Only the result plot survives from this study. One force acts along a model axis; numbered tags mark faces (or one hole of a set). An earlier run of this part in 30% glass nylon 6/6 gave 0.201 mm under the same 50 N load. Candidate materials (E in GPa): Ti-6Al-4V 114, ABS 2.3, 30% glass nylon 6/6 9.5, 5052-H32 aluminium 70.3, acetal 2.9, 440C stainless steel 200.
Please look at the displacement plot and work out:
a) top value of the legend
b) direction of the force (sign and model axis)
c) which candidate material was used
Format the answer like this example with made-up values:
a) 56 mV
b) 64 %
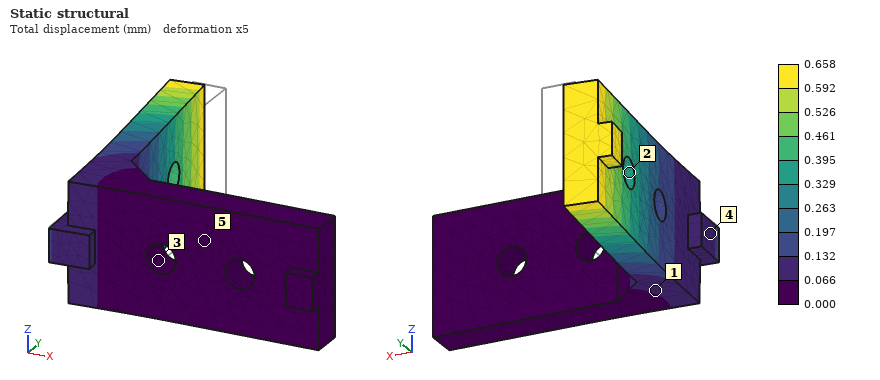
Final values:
a) 0.658 mm
b) -X
c) acetal
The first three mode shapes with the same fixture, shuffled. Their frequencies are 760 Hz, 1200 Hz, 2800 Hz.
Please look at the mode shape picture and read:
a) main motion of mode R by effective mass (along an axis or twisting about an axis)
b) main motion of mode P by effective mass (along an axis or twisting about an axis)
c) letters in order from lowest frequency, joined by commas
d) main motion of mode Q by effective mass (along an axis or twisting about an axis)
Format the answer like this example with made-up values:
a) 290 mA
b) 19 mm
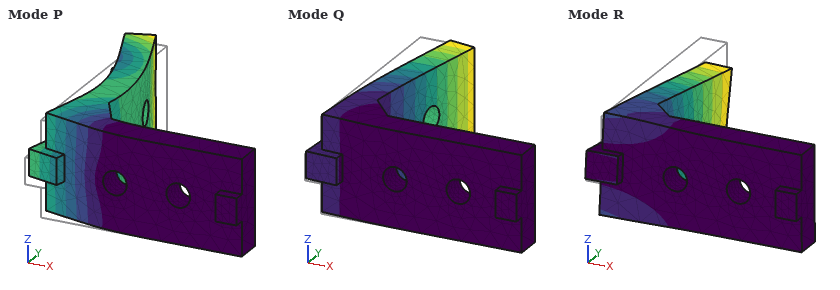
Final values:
a) along Z
b) along Y
c) Q, R, P
d) along X
